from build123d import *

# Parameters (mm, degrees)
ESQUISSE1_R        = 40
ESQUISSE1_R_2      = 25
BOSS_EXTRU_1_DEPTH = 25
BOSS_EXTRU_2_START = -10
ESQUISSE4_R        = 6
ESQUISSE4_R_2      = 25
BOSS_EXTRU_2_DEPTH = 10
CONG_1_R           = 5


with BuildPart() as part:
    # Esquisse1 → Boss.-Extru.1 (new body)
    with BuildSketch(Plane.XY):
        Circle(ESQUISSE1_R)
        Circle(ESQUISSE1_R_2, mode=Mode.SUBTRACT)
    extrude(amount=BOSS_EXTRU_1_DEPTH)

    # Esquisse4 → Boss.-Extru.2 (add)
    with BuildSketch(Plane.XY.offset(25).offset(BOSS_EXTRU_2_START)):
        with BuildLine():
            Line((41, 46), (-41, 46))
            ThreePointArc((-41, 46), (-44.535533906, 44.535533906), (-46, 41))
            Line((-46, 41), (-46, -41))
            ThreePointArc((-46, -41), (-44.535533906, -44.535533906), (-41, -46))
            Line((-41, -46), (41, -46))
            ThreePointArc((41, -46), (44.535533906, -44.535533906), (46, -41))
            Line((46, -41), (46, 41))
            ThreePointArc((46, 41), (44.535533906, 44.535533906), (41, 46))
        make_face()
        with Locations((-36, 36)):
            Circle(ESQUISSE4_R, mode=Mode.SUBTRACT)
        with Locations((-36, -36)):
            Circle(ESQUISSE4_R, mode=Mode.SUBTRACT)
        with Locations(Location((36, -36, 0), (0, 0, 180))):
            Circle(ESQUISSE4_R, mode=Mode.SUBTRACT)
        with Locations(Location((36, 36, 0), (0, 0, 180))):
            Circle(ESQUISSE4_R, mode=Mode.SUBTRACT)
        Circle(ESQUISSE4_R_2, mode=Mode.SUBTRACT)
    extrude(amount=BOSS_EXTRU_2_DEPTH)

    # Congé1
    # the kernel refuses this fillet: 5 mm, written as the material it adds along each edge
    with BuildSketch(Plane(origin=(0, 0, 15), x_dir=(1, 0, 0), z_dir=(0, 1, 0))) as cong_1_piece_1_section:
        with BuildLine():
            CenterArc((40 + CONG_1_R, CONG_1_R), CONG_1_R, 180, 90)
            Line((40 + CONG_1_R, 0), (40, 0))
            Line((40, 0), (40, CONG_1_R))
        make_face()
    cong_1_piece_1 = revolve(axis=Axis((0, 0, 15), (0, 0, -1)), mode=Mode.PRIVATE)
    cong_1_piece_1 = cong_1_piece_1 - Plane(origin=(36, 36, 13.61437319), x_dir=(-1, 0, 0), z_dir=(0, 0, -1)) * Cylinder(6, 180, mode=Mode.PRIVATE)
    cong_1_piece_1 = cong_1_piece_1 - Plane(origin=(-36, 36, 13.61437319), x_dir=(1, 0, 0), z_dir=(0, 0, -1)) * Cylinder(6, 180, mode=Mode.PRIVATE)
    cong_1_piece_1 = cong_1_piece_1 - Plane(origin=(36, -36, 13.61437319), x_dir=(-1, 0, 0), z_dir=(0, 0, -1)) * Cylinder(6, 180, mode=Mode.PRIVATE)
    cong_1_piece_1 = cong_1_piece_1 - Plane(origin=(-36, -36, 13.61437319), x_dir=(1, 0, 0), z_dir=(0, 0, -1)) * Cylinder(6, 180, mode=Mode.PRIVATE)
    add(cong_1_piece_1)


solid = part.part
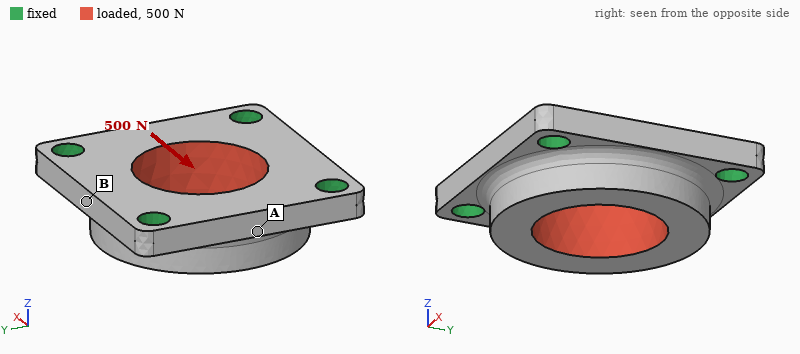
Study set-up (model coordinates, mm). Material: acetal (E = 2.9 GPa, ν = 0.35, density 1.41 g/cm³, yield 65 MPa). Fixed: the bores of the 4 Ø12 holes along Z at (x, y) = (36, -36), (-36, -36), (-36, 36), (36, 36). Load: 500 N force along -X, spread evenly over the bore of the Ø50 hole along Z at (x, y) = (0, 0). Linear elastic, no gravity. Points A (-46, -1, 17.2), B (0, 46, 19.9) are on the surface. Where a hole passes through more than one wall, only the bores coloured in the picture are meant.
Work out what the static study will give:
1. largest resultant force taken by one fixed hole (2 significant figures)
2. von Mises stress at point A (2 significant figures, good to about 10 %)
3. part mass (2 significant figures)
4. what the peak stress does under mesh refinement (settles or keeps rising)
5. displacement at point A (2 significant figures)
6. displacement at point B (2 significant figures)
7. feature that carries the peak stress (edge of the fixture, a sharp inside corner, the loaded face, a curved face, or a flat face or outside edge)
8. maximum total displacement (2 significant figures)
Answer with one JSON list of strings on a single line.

["130 N", "0.34 MPa", "150 g", "keeps rising", "6.3 µm", "2.6 µm", "edge of the fixture", "9.4 µm"]
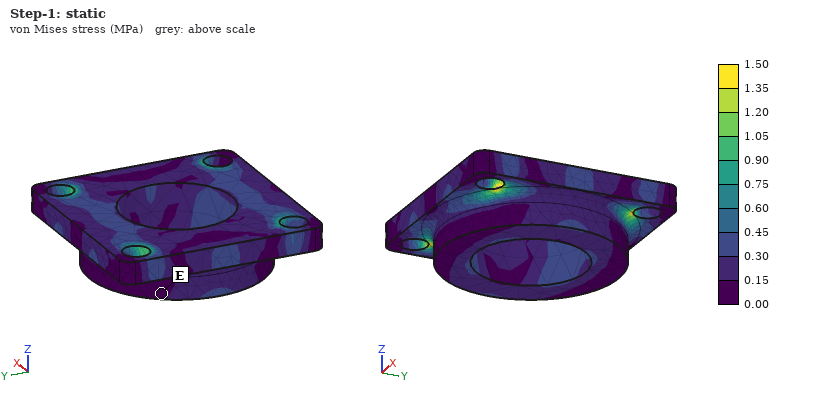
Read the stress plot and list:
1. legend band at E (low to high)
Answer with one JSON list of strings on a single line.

["0.00 to 0.15 MPa"]
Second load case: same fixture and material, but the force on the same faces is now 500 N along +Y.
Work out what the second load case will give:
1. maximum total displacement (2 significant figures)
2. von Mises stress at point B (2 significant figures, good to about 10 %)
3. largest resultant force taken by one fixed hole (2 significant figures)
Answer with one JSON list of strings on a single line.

["9.3 µm", "0.33 MPa", "130 N"]
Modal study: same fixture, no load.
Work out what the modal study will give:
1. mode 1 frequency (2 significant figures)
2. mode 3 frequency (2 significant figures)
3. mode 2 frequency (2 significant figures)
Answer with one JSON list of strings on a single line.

["3200 Hz", "3700 Hz", "3200 Hz"]
